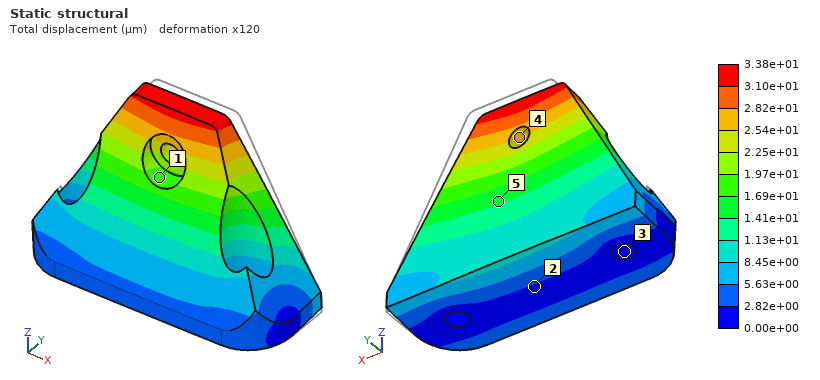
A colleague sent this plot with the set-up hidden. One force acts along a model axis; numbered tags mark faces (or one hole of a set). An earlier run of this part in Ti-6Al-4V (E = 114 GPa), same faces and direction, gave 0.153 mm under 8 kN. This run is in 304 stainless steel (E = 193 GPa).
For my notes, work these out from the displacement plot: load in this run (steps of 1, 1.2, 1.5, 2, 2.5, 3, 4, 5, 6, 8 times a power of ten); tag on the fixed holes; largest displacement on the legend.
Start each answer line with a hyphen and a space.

- 3 kN
- 3
- 3.38e+01 µm
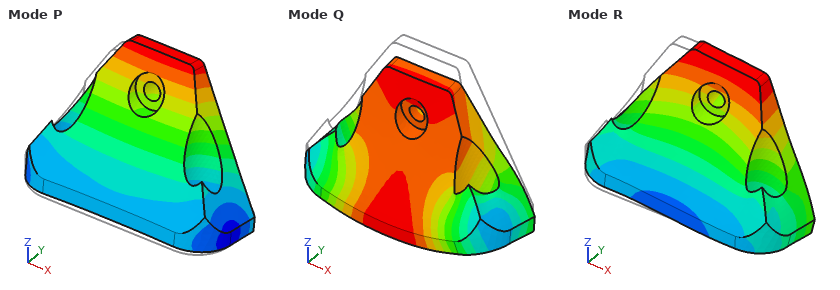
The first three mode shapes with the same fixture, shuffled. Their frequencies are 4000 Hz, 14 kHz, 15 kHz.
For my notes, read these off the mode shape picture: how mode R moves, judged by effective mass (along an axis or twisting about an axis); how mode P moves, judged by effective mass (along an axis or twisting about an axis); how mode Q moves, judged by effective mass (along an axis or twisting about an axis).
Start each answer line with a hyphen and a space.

- along X
- along Y
- along Z
